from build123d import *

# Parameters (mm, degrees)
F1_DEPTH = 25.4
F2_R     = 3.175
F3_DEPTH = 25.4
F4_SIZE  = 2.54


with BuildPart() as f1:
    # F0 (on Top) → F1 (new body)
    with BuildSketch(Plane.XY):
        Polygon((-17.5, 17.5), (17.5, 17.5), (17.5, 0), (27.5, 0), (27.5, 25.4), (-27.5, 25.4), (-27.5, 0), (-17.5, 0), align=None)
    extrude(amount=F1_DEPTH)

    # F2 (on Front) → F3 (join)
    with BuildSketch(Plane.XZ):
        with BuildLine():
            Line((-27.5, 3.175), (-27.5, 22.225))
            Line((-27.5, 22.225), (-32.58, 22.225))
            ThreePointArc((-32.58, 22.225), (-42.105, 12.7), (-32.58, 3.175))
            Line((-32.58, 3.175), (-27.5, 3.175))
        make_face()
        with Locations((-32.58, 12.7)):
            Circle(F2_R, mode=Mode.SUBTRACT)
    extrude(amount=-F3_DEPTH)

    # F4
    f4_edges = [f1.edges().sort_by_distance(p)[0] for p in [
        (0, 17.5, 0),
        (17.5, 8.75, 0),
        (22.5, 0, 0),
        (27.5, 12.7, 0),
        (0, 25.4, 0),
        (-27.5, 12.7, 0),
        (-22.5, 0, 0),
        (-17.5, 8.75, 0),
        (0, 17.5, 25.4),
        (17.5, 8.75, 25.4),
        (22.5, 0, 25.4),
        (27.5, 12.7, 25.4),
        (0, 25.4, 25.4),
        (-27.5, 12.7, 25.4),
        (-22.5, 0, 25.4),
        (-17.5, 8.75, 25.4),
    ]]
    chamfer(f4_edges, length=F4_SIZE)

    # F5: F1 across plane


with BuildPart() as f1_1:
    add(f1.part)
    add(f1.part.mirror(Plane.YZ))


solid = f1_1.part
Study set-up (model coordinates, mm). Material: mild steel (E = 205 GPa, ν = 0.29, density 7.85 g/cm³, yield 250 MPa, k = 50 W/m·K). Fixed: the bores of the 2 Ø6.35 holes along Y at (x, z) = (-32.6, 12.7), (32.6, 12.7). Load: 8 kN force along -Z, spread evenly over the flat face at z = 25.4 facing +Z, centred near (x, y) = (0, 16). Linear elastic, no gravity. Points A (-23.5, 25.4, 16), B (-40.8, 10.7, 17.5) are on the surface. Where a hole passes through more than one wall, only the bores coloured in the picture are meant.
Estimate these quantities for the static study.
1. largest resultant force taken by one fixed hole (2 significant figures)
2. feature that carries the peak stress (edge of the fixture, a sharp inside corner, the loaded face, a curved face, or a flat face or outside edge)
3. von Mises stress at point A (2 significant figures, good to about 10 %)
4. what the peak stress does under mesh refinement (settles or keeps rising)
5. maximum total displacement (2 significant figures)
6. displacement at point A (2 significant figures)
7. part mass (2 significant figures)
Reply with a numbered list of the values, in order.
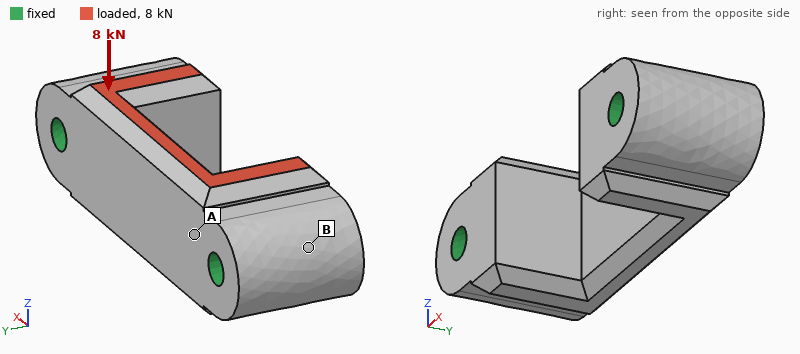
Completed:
1. 4.0 kN
2. edge of the fixture
3. 25 MPa
4. keeps rising
5. 6.6 µm
6. 2.4 µm
7. 230 g
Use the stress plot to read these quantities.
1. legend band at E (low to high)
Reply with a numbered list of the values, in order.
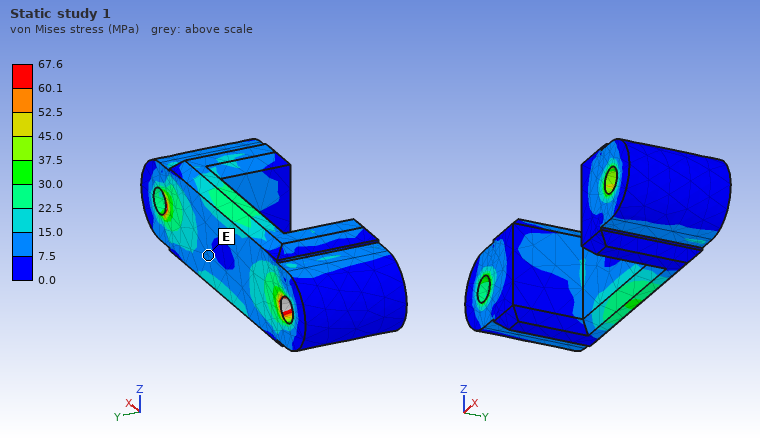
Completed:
1. 7.5 to 15.0 MPa
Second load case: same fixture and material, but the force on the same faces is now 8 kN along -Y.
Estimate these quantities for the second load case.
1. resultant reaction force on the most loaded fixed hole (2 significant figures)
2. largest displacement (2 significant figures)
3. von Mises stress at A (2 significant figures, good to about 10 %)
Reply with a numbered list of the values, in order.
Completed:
1. 4.1 kN
2. 18 µm
3. 42 MPa
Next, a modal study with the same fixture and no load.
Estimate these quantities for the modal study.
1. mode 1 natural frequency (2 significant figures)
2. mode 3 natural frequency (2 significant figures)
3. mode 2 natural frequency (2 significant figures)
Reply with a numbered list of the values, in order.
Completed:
1. 17 kHz
2. 25 kHz
3. 17 kHz
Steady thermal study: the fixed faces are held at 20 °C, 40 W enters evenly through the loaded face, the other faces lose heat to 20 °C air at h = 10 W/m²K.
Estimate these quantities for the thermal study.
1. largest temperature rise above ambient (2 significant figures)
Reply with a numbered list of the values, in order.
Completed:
1. 27 K
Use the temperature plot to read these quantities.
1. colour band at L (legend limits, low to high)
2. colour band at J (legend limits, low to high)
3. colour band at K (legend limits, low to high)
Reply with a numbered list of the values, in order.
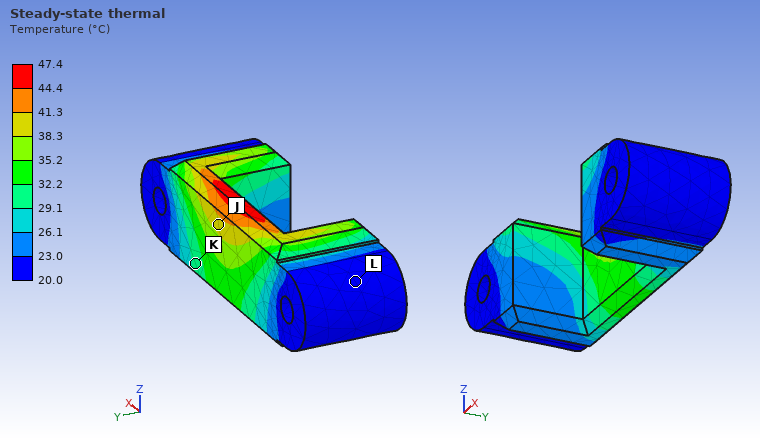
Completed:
1. 20.0 to 23.0 °C
2. 38.3 to 41.3 °C
3. 29.1 to 32.2 °C
